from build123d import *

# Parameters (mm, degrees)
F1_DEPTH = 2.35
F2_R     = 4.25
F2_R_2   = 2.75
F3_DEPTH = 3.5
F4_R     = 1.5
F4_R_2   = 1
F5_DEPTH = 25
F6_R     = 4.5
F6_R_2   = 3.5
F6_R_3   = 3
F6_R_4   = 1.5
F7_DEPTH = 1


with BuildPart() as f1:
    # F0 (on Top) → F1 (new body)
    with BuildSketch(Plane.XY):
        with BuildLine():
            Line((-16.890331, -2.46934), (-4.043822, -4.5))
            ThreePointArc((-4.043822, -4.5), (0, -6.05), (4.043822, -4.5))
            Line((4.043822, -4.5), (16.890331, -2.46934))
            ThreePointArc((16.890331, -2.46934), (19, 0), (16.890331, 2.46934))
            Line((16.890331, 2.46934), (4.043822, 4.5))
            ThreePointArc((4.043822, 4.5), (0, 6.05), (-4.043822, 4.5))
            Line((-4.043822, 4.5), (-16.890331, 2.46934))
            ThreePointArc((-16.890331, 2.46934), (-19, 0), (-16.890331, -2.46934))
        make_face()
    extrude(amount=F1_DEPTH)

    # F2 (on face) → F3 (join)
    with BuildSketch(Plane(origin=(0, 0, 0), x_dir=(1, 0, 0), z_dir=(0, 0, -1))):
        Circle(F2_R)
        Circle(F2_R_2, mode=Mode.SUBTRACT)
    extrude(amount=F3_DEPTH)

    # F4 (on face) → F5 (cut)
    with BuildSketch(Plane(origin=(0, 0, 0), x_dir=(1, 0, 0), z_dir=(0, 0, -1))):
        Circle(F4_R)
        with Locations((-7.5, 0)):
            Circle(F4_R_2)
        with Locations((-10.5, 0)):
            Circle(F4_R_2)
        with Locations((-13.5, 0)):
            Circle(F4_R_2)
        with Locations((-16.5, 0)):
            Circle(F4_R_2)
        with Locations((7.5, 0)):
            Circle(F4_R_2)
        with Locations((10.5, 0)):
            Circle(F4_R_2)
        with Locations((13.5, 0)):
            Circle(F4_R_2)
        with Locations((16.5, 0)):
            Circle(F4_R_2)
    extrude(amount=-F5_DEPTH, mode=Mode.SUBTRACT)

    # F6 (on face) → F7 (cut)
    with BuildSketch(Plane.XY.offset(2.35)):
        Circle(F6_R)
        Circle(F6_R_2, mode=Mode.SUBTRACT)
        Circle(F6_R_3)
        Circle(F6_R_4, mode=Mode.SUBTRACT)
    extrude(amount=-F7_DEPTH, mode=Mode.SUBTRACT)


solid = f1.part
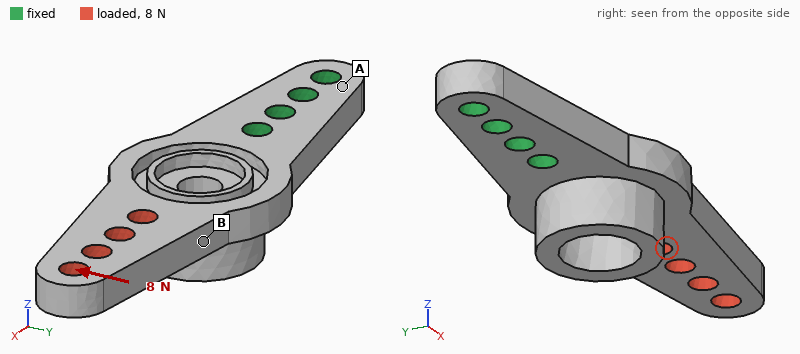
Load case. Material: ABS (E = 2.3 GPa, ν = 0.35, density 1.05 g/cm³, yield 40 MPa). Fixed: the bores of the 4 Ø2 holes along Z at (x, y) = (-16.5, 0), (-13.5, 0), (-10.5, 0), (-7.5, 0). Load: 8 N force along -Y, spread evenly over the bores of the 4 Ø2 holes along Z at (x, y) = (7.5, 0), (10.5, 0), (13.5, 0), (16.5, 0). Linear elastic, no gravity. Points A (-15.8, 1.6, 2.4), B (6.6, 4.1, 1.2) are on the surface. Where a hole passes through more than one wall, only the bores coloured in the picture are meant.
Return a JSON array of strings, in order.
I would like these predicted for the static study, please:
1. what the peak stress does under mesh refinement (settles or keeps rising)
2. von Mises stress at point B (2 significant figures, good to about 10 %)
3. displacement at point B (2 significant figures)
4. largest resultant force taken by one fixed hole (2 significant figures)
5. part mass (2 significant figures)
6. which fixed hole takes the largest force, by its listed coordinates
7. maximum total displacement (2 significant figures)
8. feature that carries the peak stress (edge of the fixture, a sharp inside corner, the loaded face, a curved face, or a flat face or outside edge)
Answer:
["keeps rising", "2.1 MPa", "0.091 mm", "28 N", "0.70 g", "(-7.5, 0)", "0.19 mm", "edge of the fixture"]
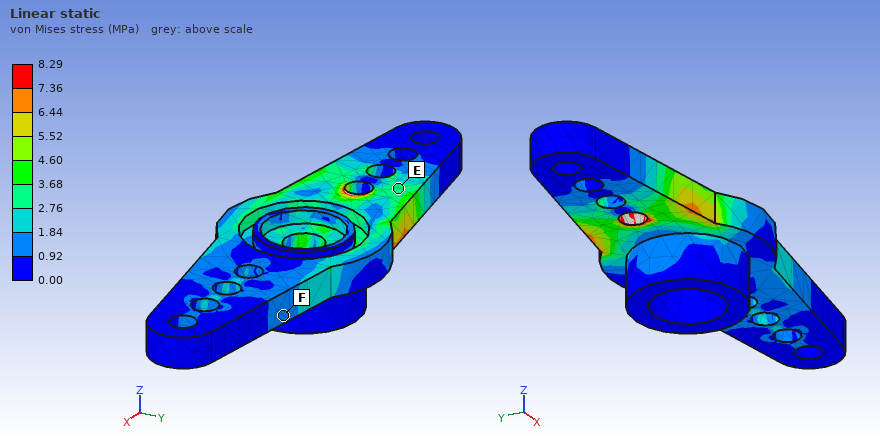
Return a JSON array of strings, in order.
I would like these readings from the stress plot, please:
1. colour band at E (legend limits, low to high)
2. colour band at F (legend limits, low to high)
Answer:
["2.76 to 3.68 MPa", "0.92 to 1.84 MPa"]
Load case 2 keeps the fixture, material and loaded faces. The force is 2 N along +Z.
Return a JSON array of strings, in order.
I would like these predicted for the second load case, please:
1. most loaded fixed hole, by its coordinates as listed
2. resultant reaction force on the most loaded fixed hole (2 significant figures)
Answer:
["(-7.5, 0)", "5.4 N"]
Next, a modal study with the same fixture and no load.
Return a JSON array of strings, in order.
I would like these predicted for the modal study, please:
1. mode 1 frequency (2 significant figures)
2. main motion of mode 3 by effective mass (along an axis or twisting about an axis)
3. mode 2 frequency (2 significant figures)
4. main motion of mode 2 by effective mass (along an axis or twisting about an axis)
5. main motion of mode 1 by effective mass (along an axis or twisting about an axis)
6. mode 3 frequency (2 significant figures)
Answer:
["990 Hz", "along Z", "2700 Hz", "along Y", "along Z", "4500 Hz"]
